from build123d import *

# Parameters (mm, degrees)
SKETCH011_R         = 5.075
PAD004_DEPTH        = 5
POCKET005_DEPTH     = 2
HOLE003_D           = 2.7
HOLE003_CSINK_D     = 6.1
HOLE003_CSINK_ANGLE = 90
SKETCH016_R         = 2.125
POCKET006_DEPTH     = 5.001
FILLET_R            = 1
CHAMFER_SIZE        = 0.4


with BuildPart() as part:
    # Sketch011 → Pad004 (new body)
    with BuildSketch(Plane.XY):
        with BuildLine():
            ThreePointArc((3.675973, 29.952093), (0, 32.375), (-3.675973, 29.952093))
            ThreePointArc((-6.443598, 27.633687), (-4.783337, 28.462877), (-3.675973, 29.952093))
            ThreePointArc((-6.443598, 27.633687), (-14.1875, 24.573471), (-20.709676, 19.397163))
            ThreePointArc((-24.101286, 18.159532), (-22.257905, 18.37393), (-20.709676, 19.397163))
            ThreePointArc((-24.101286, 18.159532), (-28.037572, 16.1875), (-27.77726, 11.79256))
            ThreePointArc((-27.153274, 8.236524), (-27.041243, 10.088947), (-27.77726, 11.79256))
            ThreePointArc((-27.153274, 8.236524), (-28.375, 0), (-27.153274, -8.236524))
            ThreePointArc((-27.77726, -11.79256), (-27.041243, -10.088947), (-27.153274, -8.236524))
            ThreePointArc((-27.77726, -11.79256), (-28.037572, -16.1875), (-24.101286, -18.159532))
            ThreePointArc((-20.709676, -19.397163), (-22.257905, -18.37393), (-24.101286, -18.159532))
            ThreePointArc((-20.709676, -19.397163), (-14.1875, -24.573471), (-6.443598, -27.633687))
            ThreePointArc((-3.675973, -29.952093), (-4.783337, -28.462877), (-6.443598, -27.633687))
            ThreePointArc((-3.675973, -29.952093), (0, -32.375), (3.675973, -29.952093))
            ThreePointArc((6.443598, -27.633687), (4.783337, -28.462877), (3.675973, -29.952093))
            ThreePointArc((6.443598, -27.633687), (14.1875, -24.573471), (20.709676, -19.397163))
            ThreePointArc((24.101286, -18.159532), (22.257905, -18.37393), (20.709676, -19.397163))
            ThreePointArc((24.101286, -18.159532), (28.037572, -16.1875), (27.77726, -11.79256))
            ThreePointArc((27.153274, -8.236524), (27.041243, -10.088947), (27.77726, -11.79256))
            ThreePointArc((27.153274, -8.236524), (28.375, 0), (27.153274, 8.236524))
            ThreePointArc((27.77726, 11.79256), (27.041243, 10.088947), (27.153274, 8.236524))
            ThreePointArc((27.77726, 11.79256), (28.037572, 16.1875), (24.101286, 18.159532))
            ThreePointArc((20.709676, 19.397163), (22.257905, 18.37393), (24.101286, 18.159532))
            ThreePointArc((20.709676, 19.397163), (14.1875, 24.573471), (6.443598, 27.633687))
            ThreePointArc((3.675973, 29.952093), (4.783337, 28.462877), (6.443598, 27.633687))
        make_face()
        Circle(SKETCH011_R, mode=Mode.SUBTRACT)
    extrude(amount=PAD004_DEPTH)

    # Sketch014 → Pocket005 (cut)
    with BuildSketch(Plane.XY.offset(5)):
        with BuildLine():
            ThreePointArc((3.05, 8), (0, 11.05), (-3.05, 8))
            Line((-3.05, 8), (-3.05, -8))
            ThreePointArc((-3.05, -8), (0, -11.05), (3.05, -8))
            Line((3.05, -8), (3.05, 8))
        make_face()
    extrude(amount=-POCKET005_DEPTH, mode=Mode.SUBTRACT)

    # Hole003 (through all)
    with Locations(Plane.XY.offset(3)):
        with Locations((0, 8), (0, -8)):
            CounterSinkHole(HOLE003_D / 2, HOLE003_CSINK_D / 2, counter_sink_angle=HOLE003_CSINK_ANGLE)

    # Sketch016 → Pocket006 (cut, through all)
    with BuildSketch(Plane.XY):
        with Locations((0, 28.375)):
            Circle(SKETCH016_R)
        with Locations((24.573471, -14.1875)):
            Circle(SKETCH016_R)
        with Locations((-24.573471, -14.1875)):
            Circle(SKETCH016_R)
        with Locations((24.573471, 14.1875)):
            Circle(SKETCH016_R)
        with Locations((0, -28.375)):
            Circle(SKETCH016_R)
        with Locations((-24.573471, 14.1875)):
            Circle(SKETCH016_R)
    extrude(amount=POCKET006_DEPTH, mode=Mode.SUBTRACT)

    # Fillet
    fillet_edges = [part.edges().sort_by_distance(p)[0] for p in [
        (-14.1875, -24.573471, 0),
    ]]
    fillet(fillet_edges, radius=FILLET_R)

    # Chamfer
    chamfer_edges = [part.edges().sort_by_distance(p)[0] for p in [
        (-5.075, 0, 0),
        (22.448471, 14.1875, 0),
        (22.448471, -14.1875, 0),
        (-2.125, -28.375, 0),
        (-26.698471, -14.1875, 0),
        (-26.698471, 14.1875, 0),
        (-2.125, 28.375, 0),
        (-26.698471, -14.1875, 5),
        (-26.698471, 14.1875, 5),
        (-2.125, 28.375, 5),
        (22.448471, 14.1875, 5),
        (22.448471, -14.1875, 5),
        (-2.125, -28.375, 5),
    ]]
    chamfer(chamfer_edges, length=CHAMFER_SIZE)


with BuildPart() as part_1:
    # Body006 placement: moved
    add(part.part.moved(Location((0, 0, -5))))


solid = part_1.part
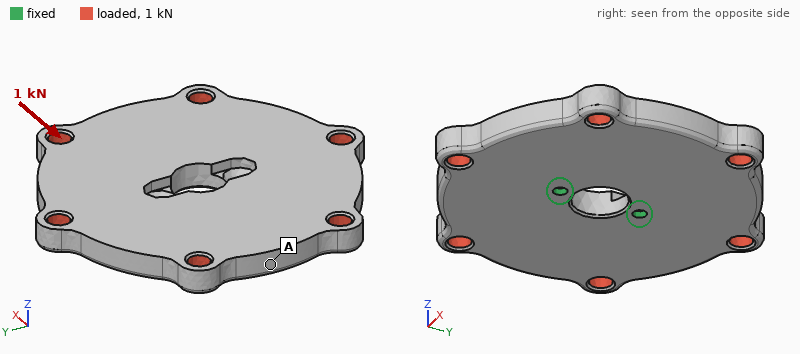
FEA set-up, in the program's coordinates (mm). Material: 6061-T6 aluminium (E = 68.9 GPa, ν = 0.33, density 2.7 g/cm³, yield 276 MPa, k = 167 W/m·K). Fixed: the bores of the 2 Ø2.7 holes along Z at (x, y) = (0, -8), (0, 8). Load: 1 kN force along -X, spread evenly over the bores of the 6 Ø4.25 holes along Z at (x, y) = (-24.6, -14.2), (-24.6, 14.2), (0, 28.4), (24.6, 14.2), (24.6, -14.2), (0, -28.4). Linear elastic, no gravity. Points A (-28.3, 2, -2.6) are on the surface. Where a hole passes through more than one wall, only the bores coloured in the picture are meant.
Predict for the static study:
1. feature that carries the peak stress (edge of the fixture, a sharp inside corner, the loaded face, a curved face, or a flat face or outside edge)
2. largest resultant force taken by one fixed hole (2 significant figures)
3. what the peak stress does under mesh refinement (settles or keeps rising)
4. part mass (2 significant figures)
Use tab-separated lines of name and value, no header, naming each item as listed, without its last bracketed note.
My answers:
feature that carries the peak stress	edge of the fixture
largest resultant force taken by one fixed hole	500 N
what the peak stress does under mesh refinement	keeps rising
part mass	33 g
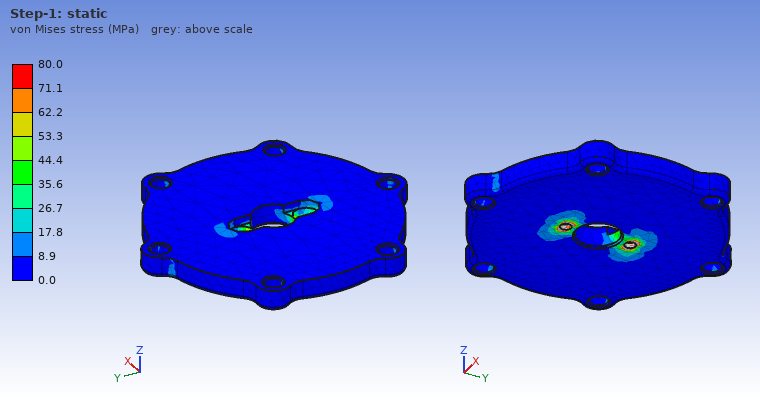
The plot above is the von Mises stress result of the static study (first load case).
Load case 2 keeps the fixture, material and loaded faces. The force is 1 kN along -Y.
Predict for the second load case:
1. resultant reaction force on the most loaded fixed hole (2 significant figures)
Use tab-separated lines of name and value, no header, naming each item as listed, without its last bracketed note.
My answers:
resultant reaction force on the most loaded fixed hole	510 N
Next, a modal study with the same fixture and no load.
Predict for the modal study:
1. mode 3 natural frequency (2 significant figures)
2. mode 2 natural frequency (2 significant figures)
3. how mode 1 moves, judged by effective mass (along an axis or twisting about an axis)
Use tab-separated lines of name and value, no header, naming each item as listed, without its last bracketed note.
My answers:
mode 3 natural frequency	4900 Hz
mode 2 natural frequency	4900 Hz
how mode 1 moves, judged by effective mass	twisting about Y
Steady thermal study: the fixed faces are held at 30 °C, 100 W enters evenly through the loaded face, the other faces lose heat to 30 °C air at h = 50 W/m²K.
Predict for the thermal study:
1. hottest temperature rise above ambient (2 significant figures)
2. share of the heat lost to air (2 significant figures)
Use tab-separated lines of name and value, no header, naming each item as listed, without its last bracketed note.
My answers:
hottest temperature rise above ambient	62 K
share of the heat lost to air	13 %
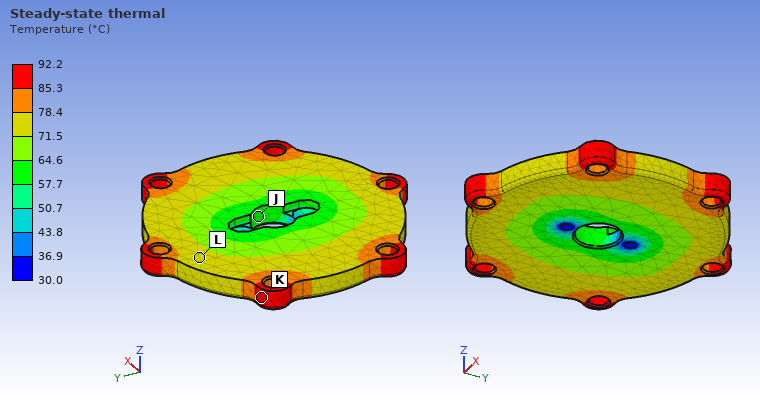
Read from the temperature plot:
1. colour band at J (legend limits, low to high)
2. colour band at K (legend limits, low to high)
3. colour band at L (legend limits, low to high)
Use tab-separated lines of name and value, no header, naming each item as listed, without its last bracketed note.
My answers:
colour band at J	57.7 to 64.6 °C
colour band at K	85.3 to 92.2 °C
colour band at L	71.5 to 78.4 °C
